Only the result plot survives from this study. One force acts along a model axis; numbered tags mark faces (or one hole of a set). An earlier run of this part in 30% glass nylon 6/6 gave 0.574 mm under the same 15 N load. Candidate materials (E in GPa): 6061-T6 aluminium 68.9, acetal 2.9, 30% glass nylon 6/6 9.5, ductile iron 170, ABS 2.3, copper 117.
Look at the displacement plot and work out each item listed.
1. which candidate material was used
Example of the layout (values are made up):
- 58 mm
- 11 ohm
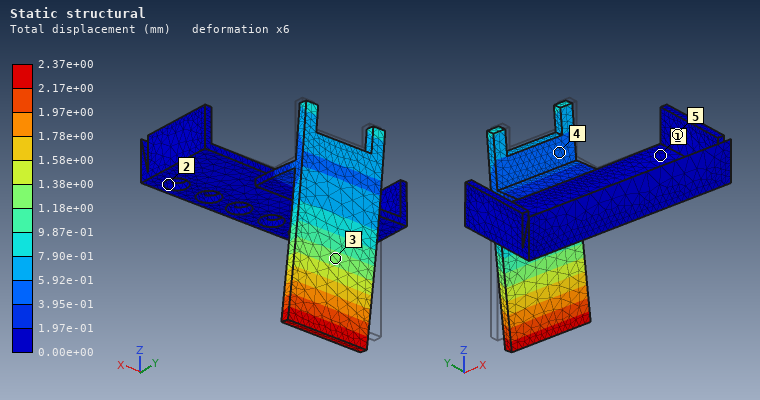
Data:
- ABS
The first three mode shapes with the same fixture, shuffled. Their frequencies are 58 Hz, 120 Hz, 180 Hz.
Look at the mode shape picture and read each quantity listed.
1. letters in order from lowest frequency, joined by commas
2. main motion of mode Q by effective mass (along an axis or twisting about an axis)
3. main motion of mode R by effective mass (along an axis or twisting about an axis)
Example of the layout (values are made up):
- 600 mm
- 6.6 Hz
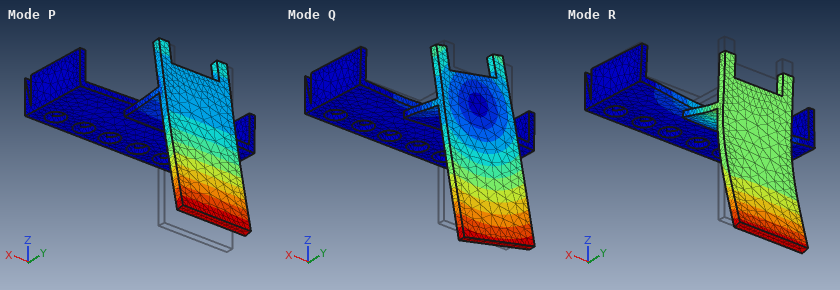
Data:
- P, Q, R
- along X
- along Z
